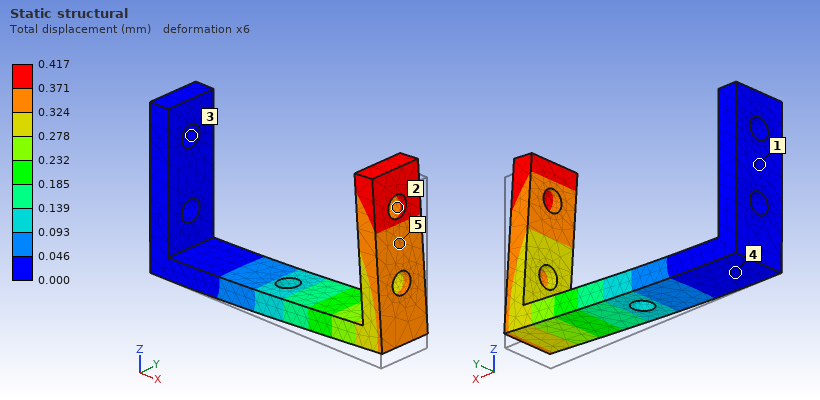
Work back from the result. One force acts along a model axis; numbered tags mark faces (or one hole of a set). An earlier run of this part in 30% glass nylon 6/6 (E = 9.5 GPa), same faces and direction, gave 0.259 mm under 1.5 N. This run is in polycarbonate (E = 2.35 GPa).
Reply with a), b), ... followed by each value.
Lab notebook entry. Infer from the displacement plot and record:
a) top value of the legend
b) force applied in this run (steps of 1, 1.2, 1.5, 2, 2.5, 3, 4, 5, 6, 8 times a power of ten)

a) 0.417 mm
b) 0.6 N
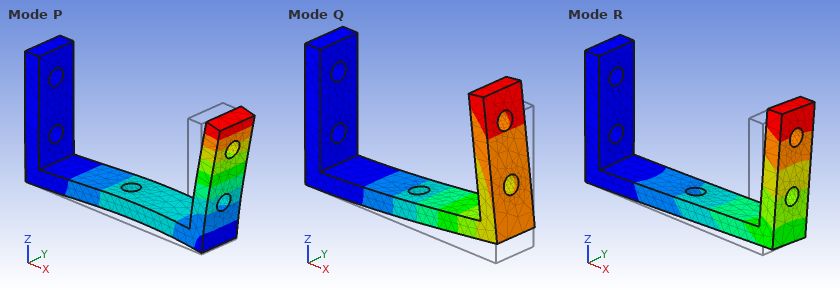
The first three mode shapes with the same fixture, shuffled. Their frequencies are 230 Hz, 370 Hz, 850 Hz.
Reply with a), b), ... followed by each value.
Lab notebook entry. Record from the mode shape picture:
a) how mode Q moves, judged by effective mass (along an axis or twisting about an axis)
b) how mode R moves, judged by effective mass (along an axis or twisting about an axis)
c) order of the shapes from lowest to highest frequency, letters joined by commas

a) along Z
b) along Y
c) Q, R, P
